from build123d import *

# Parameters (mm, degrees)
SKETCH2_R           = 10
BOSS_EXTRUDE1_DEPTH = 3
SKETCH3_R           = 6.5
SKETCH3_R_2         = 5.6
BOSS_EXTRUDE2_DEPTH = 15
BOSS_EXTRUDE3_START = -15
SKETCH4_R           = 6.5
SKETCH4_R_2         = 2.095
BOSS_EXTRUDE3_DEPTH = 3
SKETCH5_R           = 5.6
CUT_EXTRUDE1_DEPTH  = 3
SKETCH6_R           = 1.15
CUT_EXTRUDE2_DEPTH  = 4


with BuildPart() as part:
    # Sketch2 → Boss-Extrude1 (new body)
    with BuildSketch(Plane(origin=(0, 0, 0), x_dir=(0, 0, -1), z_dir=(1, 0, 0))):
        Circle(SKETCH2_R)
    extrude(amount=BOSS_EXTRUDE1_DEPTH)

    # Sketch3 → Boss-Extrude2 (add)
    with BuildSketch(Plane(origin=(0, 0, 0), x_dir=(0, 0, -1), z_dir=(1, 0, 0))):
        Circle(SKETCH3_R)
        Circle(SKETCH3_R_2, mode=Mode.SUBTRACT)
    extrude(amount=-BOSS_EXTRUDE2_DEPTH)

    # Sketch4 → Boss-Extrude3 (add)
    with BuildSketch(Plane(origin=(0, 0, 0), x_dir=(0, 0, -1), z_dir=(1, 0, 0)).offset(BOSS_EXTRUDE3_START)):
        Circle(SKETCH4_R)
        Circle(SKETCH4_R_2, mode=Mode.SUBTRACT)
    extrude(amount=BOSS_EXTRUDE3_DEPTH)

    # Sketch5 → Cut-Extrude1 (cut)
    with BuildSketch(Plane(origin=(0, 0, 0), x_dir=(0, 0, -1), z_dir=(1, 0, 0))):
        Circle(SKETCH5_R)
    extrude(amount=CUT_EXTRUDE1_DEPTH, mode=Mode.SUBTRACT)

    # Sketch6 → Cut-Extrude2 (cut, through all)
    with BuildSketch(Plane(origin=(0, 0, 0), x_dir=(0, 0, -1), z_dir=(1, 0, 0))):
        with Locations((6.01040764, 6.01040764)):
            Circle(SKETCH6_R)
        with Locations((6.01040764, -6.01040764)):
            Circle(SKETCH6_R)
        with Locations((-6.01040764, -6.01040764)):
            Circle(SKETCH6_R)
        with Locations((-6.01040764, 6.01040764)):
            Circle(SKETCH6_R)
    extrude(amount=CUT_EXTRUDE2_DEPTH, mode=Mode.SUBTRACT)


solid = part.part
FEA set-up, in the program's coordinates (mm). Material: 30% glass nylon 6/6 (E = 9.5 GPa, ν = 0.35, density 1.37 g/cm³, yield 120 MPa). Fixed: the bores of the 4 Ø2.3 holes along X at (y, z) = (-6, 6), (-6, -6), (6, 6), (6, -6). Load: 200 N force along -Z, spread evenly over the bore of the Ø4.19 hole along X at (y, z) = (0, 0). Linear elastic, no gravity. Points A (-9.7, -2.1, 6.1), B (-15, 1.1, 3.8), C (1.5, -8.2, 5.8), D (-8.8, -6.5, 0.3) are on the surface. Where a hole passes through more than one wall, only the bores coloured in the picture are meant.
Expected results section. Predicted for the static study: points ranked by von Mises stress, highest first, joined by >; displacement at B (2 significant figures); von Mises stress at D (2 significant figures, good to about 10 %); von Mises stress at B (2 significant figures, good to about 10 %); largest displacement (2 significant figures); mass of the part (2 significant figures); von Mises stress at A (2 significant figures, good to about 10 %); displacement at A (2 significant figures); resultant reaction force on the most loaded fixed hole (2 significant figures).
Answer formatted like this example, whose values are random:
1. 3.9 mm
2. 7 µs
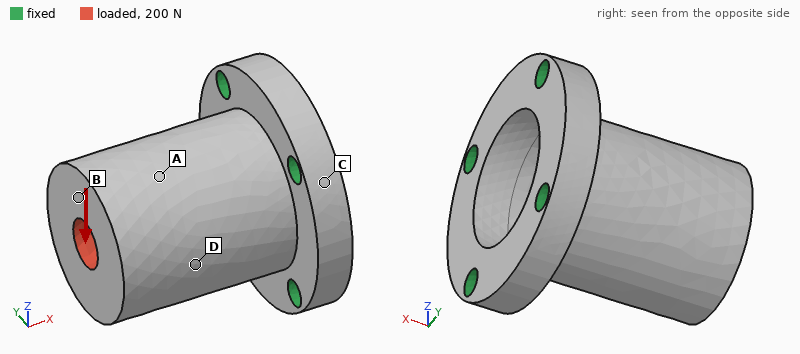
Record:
1. D > A > B > C
2. 0.11 mm
3. 18 MPa
4. 6.0 MPa
5. 0.11 mm
6. 1.9 g
7. 12 MPa
8. 0.076 mm
9. 150 N
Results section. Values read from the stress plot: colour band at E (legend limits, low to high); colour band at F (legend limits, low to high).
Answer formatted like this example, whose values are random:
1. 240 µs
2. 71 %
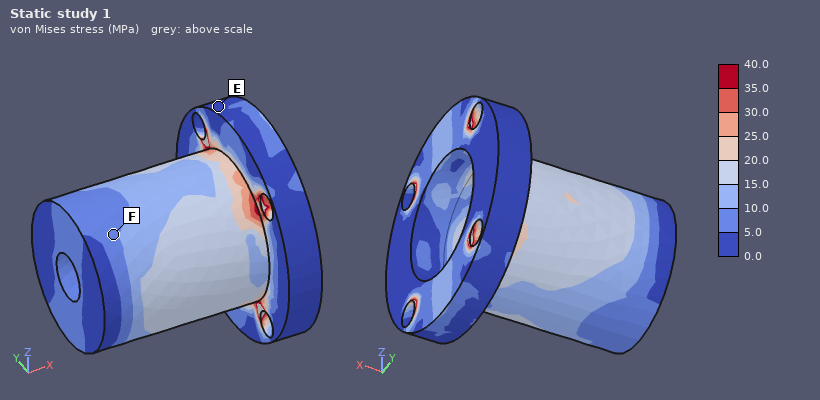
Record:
1. 0.0 to 5.0 MPa
2. 5.0 to 10.0 MPa
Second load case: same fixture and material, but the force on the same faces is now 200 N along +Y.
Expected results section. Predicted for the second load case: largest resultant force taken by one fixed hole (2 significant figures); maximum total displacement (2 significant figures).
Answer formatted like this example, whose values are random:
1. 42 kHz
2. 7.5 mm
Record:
1. 150 N
2. 0.11 mm
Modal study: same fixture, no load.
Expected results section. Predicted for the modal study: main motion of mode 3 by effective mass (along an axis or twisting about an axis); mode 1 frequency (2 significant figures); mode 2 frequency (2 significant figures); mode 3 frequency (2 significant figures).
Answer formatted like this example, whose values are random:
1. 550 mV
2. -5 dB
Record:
1. twisting about X
2. 8900 Hz
3. 8900 Hz
4. 21 kHz
